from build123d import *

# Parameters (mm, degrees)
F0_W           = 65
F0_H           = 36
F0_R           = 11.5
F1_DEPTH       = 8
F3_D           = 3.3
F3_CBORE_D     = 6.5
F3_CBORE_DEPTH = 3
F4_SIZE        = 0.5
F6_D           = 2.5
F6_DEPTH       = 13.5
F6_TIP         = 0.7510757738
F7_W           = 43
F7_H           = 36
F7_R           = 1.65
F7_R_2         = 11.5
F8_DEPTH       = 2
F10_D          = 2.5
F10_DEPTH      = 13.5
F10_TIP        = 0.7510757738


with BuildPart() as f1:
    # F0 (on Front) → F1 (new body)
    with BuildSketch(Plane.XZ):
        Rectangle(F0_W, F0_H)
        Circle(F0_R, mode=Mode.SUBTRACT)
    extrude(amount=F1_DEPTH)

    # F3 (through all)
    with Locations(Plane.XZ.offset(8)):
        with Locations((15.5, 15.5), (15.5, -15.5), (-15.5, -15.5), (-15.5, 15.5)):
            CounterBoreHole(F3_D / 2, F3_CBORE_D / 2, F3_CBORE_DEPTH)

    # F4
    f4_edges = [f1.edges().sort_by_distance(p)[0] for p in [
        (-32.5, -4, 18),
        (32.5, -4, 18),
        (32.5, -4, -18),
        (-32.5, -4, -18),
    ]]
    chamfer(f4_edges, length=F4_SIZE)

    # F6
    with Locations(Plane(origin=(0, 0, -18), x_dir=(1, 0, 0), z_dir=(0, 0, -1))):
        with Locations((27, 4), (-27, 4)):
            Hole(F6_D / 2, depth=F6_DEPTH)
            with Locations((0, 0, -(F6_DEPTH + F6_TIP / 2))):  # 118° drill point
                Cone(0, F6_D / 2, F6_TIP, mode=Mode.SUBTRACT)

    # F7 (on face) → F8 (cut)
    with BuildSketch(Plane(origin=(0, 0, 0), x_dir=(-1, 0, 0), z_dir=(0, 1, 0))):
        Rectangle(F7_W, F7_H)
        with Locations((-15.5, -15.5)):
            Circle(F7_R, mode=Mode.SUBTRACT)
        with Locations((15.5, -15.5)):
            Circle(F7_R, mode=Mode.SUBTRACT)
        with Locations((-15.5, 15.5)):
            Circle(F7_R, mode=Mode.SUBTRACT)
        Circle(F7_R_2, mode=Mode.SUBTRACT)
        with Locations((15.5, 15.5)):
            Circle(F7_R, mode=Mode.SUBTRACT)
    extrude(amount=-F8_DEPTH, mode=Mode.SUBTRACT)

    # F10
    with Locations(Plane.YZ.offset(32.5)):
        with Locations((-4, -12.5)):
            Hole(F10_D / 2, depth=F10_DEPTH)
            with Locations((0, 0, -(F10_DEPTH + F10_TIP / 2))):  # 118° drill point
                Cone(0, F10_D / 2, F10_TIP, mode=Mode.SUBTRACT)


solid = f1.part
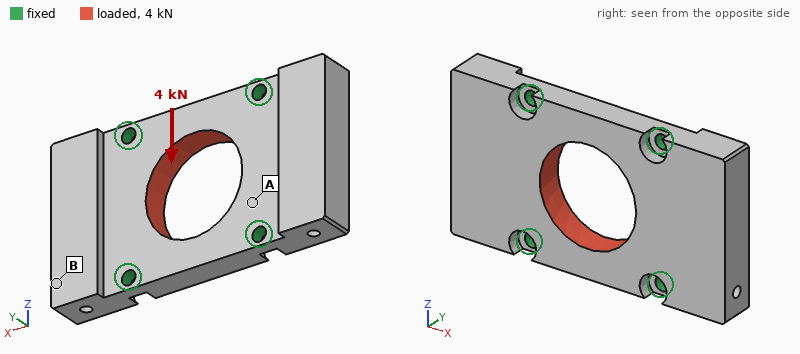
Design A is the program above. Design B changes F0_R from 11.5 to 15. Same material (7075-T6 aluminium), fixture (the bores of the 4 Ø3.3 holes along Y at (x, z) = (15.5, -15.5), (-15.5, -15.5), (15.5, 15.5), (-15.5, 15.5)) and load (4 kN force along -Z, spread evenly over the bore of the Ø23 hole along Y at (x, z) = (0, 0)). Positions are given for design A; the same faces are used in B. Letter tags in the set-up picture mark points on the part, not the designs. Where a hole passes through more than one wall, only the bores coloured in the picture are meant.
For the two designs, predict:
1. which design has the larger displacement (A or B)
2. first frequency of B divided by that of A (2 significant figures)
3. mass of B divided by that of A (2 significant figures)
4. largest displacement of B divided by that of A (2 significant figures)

B
0.90
0.86
2.0
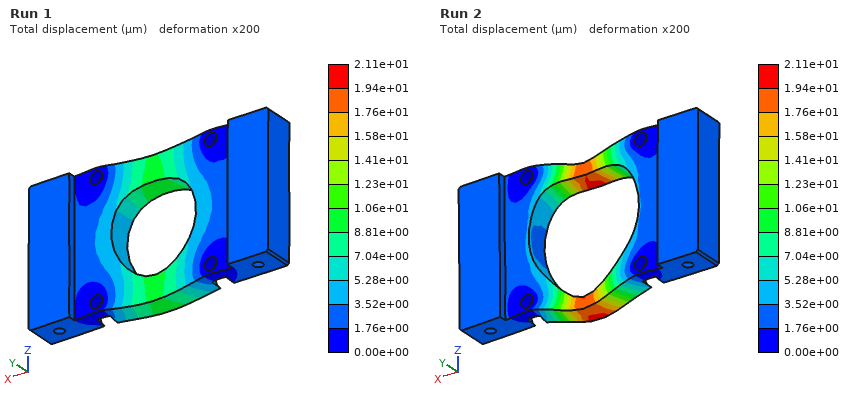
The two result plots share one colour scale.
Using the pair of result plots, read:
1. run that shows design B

Run 2
